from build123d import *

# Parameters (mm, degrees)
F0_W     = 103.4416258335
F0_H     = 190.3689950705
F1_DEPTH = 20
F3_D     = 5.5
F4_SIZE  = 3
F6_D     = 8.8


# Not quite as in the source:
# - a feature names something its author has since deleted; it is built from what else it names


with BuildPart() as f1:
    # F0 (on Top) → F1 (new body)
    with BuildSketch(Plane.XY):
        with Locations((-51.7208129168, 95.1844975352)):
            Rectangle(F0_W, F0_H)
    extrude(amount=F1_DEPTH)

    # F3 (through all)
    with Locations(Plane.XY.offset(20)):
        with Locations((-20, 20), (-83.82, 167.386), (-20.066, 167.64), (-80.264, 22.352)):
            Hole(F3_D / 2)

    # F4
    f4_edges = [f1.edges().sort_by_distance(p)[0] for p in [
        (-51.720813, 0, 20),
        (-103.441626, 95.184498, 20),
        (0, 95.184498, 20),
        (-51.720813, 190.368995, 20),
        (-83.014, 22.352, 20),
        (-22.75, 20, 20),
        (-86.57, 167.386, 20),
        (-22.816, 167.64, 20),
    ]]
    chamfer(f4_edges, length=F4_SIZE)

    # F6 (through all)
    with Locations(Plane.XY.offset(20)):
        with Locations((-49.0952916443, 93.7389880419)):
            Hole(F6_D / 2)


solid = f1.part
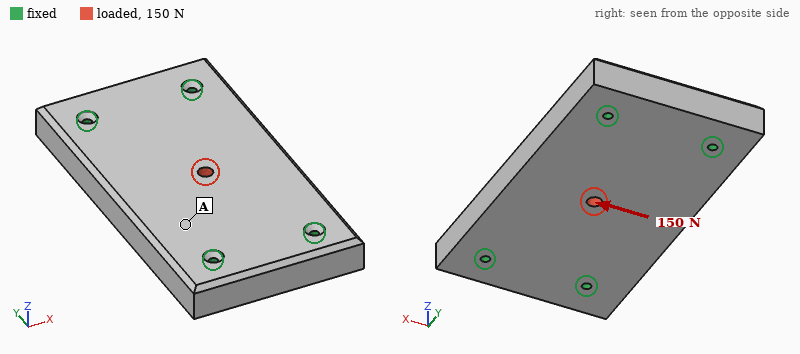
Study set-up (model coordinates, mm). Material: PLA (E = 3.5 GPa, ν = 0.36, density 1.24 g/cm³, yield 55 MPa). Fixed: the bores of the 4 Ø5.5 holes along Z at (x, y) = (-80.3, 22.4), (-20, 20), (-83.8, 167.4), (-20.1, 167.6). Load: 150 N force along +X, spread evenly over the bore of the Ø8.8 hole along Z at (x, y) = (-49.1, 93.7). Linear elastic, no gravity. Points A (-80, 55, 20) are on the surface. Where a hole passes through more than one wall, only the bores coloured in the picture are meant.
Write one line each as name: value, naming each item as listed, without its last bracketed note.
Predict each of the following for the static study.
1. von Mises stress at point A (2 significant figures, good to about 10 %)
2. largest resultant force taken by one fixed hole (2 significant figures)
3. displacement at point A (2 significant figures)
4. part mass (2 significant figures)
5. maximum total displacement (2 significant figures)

von Mises stress at point A: 0.065 MPa
largest resultant force taken by one fixed hole: 53 N
displacement at point A: 1.7 µm
part mass: 480 g
maximum total displacement: 3.9 µm
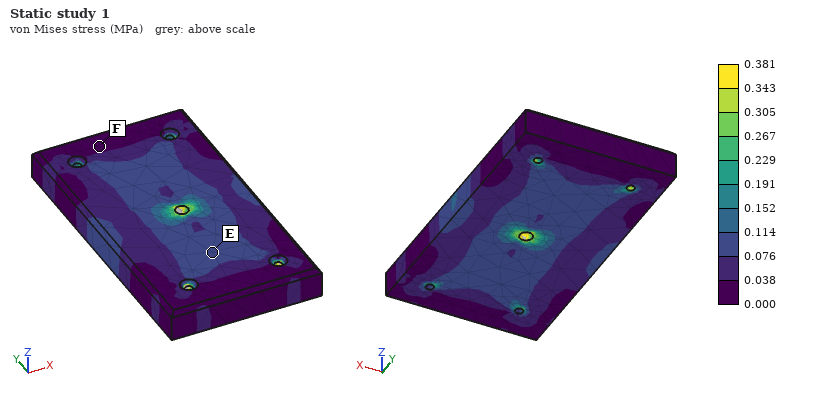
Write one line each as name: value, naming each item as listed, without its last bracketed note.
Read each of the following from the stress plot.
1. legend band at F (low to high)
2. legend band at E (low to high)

legend band at F: 0.000 to 0.038 MPa
legend band at E: 0.076 to 0.114 MPa
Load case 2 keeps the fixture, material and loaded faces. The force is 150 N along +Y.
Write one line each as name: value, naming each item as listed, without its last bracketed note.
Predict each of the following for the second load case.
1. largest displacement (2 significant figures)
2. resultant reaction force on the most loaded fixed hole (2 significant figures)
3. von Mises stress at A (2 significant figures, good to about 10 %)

largest displacement: 2.1 µm
resultant reaction force on the most loaded fixed hole: 39 N
von Mises stress at A: 0.040 MPa
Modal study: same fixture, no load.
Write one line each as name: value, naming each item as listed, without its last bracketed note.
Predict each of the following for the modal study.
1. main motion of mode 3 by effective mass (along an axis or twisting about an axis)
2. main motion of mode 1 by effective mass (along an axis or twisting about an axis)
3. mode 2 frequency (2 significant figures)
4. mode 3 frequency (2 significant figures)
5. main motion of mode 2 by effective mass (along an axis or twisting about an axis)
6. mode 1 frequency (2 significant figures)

main motion of mode 3 by effective mass: along X
main motion of mode 1 by effective mass: along Z
mode 2 frequency: 1600 Hz
mode 3 frequency: 2700 Hz
main motion of mode 2 by effective mass: twisting about Y
mode 1 frequency: 1100 Hz
